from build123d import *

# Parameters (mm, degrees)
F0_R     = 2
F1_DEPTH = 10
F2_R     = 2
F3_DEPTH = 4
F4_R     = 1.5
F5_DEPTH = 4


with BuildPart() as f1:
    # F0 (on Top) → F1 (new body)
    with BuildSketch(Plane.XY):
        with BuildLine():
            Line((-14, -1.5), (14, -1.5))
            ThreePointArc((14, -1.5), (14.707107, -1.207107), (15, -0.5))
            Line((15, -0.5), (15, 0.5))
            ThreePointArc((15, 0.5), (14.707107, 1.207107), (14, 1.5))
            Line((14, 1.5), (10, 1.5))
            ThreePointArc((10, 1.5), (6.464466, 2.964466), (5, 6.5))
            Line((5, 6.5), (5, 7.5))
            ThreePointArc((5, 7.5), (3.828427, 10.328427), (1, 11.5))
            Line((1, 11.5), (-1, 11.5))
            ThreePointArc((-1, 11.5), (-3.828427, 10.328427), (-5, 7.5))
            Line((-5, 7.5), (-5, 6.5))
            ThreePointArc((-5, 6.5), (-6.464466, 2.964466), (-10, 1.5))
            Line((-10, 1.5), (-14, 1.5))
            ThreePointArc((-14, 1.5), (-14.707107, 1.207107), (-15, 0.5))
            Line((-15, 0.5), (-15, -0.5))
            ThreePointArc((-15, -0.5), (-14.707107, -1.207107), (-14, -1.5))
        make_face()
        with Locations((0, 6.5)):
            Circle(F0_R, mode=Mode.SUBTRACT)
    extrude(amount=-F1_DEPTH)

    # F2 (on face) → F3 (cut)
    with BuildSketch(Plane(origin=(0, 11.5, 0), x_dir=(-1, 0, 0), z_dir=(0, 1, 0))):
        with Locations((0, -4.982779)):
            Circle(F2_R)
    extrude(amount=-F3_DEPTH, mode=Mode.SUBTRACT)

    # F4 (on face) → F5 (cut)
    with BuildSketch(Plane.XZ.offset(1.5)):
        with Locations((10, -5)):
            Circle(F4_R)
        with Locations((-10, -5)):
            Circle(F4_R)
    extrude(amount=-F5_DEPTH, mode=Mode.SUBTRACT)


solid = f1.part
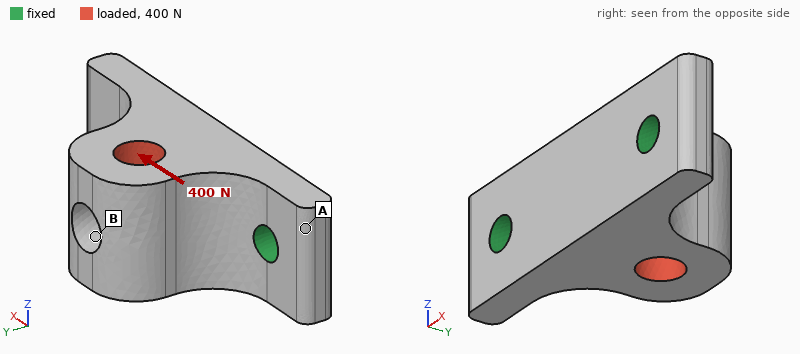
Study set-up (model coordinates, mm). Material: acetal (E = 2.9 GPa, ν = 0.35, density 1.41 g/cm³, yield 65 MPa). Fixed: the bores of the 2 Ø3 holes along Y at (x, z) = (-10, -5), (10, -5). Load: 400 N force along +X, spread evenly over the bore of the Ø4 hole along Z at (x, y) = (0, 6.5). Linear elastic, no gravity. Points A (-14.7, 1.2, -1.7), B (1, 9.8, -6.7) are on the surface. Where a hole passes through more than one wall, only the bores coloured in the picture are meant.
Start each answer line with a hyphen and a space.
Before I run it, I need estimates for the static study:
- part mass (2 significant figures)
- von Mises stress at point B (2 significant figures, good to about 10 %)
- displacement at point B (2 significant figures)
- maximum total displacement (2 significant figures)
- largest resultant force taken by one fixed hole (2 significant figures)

- 2.4 g
- 4.7 MPa
- 69 µm
- 77 µm
- 250 N
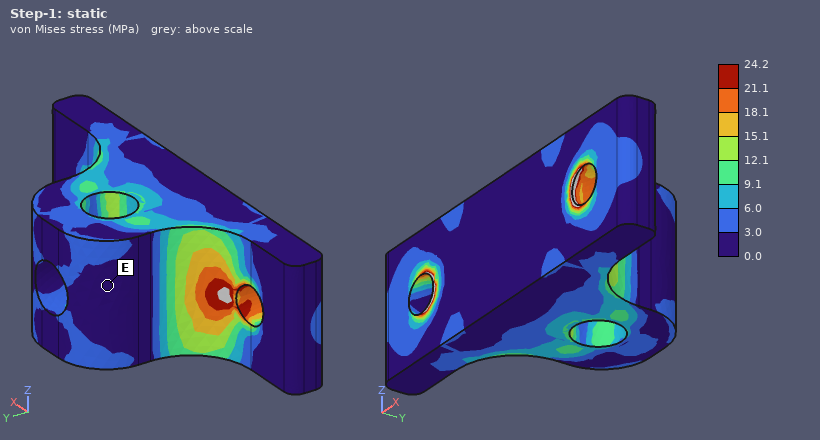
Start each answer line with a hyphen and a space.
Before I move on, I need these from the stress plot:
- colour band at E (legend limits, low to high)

- 0.0 to 3.0 MPa
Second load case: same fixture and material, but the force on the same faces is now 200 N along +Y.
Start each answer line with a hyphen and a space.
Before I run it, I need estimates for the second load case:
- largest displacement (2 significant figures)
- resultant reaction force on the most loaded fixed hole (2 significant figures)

- 33 µm
- 120 N
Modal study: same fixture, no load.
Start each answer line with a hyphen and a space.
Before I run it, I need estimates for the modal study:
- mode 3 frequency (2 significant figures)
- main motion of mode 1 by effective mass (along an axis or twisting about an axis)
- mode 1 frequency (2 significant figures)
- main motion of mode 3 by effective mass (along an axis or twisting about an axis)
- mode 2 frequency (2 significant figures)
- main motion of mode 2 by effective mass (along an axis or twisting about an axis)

- 12 kHz
- along Z
- 4900 Hz
- along X
- 10 kHz
- along Y
